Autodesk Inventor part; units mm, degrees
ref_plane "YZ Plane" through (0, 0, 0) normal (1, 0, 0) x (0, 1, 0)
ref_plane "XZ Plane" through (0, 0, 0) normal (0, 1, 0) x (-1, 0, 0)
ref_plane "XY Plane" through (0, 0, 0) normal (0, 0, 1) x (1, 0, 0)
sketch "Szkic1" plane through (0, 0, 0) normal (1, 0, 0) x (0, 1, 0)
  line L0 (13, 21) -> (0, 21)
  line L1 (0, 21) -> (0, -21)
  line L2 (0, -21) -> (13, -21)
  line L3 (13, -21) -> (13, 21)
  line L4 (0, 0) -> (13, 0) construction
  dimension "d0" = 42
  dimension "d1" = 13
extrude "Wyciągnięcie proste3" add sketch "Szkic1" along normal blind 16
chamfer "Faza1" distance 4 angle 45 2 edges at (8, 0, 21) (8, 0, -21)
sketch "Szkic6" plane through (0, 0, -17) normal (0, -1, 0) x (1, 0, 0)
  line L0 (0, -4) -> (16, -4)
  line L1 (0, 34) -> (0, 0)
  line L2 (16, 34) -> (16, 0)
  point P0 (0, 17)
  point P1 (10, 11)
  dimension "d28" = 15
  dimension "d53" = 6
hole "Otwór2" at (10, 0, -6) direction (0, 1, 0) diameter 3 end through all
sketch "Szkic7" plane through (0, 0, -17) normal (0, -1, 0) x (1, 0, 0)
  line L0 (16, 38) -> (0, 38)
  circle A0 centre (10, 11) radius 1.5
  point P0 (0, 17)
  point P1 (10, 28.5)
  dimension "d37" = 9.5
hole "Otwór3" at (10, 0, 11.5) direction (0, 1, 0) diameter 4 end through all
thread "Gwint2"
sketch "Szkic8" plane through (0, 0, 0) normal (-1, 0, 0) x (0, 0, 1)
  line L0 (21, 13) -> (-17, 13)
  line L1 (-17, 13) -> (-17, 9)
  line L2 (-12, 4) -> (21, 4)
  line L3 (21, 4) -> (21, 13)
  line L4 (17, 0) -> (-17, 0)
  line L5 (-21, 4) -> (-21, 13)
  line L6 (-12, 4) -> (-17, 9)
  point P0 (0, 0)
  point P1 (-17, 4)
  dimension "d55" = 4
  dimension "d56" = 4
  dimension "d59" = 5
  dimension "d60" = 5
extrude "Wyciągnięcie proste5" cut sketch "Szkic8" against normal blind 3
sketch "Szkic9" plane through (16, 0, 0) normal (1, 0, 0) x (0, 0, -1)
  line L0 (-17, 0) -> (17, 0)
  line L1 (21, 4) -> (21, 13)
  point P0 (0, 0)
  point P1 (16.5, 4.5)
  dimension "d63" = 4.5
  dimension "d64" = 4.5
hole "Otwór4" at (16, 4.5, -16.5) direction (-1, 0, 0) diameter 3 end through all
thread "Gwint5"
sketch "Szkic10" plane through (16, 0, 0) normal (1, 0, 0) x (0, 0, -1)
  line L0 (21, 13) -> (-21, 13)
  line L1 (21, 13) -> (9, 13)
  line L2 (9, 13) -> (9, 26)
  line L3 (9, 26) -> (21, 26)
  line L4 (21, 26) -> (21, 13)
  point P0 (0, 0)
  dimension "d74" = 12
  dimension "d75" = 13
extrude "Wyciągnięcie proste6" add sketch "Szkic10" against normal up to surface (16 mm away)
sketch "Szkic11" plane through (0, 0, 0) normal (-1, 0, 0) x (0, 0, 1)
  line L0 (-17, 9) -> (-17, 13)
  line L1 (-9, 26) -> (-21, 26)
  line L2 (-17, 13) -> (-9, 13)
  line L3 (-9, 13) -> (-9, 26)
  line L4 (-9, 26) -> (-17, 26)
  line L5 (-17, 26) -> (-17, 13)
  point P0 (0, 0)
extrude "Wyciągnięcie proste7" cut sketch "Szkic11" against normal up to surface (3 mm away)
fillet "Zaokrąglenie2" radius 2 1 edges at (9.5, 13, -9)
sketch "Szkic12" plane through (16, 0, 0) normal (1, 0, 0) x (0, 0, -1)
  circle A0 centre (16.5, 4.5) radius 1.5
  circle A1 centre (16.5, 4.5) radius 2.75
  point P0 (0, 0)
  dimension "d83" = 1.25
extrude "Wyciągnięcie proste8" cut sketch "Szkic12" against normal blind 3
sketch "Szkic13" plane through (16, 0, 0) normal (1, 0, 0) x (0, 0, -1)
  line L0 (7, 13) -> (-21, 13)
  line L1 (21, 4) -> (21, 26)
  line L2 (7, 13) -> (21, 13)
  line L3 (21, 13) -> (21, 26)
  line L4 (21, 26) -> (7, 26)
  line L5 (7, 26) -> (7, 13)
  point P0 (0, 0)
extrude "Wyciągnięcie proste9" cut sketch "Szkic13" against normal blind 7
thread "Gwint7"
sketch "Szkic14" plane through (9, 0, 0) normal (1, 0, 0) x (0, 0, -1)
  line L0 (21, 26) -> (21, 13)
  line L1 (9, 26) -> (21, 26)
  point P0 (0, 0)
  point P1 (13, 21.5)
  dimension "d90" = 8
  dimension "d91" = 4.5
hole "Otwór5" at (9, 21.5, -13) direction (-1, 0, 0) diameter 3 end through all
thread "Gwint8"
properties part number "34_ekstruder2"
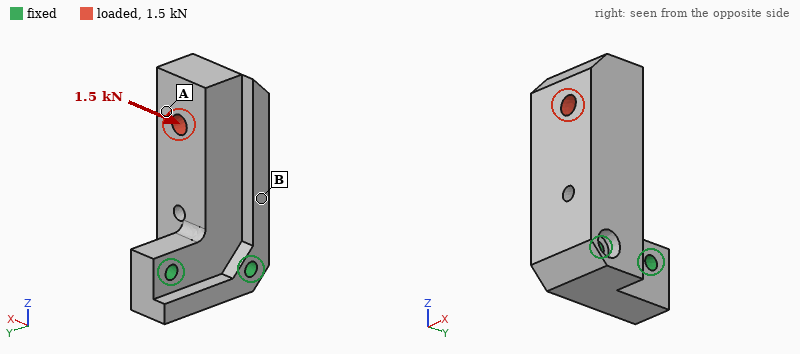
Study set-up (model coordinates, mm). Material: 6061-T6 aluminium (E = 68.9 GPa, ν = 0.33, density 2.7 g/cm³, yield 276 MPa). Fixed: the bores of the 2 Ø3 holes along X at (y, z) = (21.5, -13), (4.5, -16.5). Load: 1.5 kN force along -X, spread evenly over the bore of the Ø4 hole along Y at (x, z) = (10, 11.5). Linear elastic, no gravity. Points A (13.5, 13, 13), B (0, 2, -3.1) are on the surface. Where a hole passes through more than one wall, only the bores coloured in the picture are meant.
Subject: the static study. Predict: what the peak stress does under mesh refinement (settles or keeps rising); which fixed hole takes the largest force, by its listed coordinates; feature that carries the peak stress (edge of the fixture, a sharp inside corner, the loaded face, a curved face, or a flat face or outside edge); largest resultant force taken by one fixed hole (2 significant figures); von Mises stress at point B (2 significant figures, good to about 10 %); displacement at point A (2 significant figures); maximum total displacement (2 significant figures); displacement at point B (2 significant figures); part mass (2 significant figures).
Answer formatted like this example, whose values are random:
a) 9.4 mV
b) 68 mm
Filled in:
a) keeps rising
b) (4.5, -16.5)
c) edge of the fixture
d) 1.2 kN
e) 61 MPa
f) 0.099 mm
g) 0.13 mm
h) 0.039 mm
i) 22 g
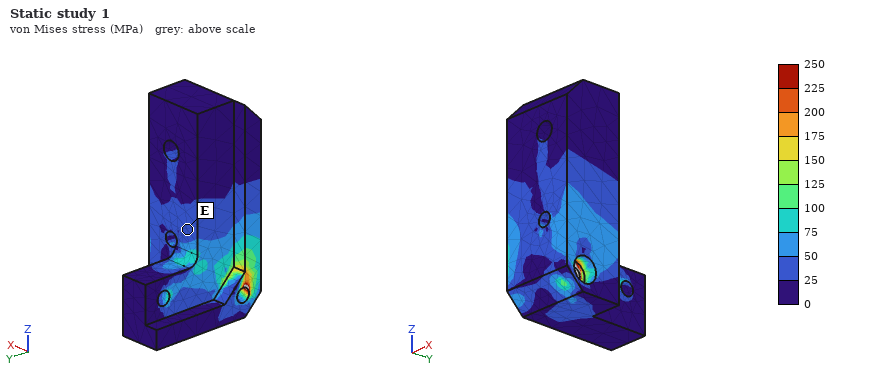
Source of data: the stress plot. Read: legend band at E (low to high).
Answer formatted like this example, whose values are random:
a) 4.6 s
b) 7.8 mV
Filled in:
a) 25 to 50 MPa
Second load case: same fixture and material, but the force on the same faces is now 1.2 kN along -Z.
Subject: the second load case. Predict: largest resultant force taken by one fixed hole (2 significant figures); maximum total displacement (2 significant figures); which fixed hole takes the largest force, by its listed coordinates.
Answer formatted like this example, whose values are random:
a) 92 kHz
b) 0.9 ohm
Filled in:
a) 1.1 kN
b) 11 µm
c) (4.5, -16.5)
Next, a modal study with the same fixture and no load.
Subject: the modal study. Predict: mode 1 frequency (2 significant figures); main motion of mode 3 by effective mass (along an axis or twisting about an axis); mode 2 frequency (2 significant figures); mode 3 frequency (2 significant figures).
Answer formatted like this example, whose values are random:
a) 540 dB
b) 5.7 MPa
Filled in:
a) 6600 Hz
b) twisting about Z
c) 6700 Hz
d) 18 kHz
